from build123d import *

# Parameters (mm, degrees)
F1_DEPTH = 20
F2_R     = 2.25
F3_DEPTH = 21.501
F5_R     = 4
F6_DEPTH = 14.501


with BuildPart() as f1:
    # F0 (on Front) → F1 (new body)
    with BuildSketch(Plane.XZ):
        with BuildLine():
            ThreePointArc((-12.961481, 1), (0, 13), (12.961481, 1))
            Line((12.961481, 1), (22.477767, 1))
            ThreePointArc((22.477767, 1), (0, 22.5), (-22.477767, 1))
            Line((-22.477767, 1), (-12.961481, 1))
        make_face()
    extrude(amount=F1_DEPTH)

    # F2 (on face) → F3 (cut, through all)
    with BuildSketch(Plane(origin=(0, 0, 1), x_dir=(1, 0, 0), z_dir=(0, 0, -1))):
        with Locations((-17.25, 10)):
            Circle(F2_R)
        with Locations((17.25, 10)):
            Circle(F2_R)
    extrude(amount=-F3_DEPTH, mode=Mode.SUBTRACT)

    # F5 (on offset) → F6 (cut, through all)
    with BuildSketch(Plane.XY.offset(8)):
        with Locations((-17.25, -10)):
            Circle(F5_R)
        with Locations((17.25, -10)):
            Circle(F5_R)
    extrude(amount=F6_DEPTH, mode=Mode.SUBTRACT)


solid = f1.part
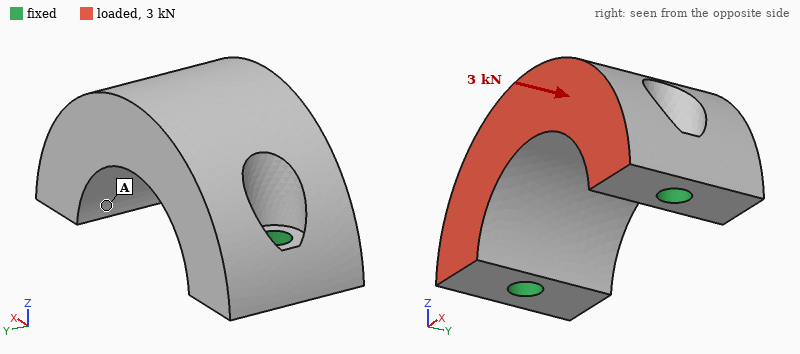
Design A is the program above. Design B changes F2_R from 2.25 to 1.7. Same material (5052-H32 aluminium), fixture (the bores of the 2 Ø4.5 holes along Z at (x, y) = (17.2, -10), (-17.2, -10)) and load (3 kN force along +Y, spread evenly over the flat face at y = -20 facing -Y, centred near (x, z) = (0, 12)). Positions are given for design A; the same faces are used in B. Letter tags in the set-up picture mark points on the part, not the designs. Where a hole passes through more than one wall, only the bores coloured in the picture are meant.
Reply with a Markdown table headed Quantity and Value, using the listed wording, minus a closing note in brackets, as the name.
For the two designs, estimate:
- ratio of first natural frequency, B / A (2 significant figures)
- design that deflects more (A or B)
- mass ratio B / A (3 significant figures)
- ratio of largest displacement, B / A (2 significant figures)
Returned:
| Quantity | Value |
|---|---|
| ratio of first natural frequency, B / A | 0.88 |
| design that deflects more | B |
| mass ratio B / A | 1.01 |
| ratio of largest displacement, B / A | 1.3 |
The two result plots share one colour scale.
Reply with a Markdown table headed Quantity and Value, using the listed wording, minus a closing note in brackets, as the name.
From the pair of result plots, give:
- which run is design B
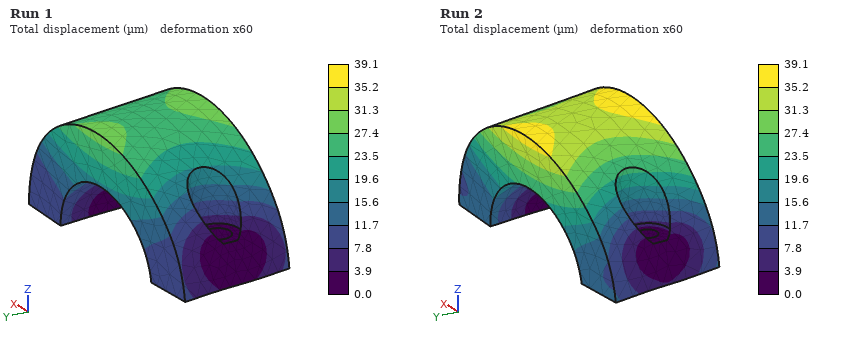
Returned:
| Quantity | Value |
|---|---|
| which run is design B | Run 2 |
